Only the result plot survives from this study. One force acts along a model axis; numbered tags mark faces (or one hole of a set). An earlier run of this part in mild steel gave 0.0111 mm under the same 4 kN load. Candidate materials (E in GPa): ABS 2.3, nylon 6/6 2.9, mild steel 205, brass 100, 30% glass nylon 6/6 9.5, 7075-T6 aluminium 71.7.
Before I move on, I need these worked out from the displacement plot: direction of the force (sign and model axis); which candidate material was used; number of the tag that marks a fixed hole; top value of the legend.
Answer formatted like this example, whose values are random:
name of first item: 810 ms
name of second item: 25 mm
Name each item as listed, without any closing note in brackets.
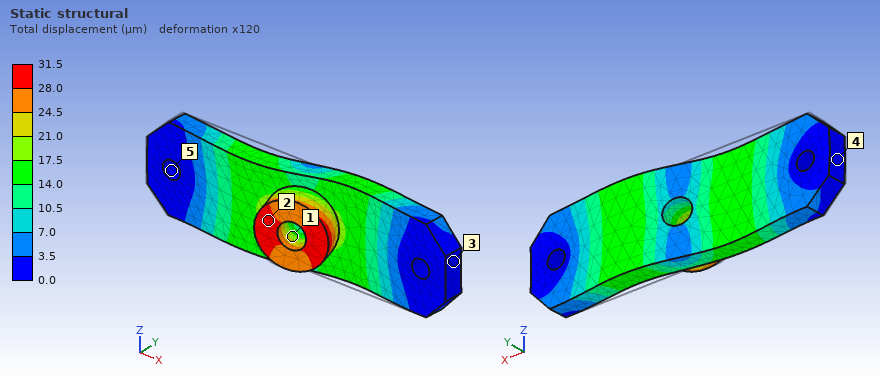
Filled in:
direction of the force: +X
which candidate material was used: 7075-T6 aluminium
number of the tag that marks a fixed hole: 5
top value of the legend: 31.5 µm
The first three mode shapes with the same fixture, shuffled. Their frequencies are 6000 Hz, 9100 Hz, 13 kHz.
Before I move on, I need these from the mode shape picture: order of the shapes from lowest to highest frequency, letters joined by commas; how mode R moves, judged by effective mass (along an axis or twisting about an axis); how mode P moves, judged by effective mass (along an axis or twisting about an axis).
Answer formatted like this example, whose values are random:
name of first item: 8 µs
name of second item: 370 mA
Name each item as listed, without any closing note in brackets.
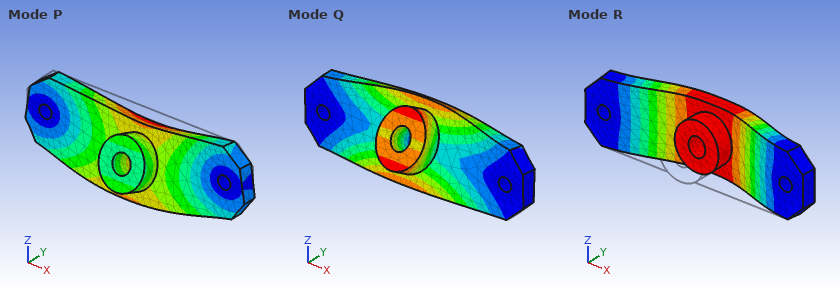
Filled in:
order of the shapes from lowest to highest frequency, letters joined by commas: R, Q, P
how mode R moves, judged by effective mass: along Y
how mode P moves, judged by effective mass: along Z
